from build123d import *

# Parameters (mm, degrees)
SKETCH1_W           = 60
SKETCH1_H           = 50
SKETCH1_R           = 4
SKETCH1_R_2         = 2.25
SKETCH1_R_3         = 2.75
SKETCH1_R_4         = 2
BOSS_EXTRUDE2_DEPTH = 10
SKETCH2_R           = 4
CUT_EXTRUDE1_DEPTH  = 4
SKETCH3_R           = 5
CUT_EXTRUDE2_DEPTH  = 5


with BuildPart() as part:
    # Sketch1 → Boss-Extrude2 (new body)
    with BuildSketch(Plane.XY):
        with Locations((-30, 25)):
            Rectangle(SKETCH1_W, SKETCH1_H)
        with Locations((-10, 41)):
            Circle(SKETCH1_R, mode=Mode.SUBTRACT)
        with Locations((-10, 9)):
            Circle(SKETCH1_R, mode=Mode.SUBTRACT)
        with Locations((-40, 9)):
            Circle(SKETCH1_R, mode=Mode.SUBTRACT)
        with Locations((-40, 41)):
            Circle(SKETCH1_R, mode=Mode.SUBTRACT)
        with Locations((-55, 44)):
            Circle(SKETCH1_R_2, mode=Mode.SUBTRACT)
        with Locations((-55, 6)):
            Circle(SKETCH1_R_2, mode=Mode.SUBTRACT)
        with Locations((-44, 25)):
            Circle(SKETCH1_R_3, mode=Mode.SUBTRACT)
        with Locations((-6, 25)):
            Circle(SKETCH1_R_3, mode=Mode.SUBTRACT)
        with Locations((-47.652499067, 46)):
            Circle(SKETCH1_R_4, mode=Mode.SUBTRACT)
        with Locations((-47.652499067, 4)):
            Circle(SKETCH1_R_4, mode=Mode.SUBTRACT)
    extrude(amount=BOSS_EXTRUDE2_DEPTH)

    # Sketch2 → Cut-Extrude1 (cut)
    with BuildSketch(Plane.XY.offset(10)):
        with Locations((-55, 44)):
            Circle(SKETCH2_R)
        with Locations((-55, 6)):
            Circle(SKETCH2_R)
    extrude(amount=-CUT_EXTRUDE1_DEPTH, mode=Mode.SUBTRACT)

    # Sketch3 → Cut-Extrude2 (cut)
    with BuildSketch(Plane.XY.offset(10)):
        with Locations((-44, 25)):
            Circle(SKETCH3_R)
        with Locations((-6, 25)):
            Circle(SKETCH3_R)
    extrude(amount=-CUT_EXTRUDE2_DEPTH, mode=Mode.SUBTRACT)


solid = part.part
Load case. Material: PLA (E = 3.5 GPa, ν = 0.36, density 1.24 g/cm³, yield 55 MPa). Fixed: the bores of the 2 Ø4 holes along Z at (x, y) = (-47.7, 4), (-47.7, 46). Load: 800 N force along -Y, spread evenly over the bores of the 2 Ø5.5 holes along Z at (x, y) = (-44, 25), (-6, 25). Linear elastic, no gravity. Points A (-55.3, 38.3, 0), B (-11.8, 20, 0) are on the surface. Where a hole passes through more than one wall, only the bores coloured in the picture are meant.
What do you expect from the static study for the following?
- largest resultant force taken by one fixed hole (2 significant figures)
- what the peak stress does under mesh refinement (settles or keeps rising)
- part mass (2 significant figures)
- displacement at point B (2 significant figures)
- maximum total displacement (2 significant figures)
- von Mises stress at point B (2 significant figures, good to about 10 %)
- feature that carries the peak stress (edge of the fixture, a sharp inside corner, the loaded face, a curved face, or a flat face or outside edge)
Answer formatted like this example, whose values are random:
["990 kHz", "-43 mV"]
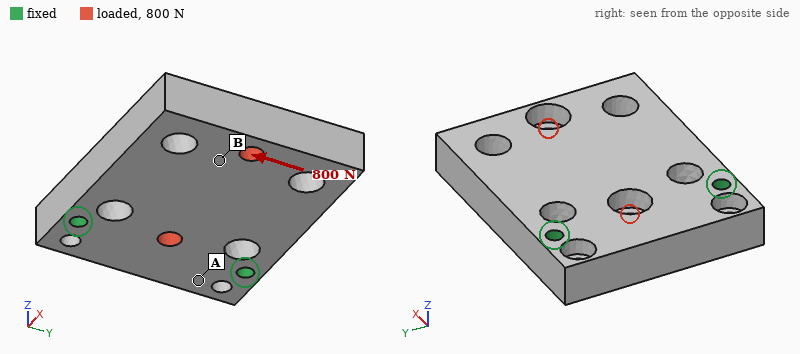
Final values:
["580 N", "keeps rising", "32 g", "0.087 mm", "0.12 mm", "4.3 MPa", "edge of the fixture"]
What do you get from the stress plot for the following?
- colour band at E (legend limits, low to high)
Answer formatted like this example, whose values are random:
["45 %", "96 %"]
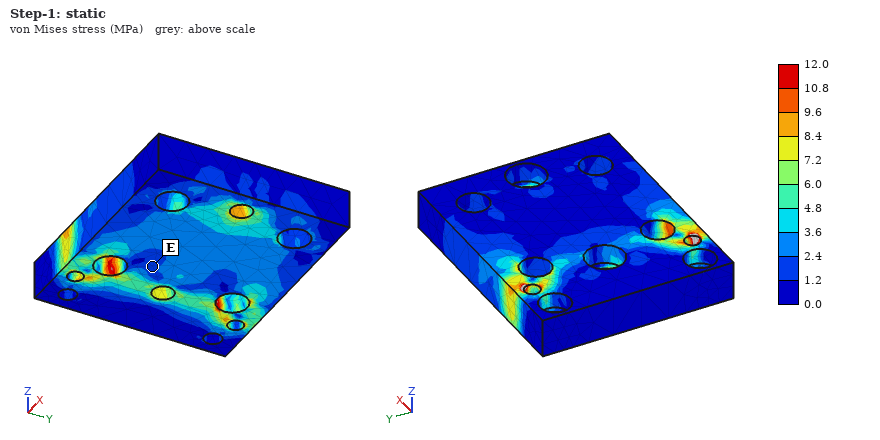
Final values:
["1.2 to 2.4 MPa"]
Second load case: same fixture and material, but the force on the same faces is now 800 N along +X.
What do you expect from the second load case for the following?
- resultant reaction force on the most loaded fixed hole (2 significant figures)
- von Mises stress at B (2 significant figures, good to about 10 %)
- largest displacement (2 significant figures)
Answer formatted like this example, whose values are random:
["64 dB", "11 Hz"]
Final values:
["400 N", "4.2 MPa", "0.20 mm"]
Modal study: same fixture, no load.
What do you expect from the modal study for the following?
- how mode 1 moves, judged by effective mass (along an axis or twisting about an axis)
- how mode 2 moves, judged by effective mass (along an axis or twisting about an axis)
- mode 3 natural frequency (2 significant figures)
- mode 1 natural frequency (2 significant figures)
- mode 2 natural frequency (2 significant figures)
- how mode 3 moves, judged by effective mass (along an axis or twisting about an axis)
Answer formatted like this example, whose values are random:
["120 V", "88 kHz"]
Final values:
["along Z", "twisting about X", "3200 Hz", "870 Hz", "2300 Hz", "along Y"]
